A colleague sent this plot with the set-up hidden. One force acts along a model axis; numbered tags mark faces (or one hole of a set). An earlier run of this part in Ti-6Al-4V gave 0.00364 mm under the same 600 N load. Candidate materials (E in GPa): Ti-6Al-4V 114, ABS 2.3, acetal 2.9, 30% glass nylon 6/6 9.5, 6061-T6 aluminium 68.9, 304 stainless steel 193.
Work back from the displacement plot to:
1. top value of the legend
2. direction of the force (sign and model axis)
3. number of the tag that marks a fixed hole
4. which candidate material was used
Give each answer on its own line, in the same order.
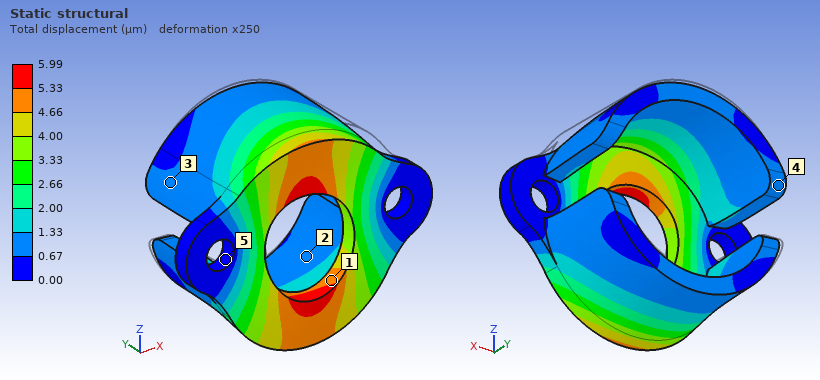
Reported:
5.99 µm
-Z
5
6061-T6 aluminium
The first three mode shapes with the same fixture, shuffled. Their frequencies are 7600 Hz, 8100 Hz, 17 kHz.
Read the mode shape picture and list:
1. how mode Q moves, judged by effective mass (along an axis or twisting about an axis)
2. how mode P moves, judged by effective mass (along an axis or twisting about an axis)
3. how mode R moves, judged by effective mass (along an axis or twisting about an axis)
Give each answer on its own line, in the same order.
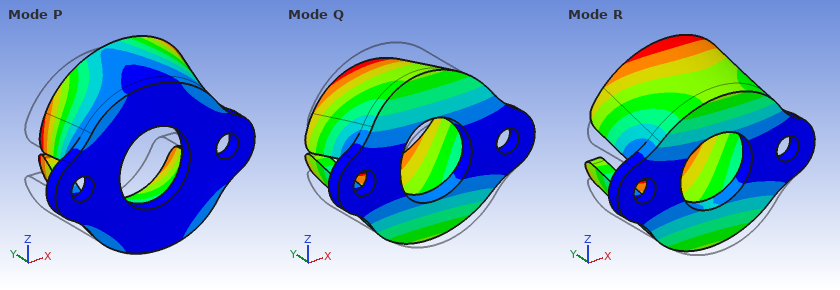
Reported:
along Y
along X
along Z
